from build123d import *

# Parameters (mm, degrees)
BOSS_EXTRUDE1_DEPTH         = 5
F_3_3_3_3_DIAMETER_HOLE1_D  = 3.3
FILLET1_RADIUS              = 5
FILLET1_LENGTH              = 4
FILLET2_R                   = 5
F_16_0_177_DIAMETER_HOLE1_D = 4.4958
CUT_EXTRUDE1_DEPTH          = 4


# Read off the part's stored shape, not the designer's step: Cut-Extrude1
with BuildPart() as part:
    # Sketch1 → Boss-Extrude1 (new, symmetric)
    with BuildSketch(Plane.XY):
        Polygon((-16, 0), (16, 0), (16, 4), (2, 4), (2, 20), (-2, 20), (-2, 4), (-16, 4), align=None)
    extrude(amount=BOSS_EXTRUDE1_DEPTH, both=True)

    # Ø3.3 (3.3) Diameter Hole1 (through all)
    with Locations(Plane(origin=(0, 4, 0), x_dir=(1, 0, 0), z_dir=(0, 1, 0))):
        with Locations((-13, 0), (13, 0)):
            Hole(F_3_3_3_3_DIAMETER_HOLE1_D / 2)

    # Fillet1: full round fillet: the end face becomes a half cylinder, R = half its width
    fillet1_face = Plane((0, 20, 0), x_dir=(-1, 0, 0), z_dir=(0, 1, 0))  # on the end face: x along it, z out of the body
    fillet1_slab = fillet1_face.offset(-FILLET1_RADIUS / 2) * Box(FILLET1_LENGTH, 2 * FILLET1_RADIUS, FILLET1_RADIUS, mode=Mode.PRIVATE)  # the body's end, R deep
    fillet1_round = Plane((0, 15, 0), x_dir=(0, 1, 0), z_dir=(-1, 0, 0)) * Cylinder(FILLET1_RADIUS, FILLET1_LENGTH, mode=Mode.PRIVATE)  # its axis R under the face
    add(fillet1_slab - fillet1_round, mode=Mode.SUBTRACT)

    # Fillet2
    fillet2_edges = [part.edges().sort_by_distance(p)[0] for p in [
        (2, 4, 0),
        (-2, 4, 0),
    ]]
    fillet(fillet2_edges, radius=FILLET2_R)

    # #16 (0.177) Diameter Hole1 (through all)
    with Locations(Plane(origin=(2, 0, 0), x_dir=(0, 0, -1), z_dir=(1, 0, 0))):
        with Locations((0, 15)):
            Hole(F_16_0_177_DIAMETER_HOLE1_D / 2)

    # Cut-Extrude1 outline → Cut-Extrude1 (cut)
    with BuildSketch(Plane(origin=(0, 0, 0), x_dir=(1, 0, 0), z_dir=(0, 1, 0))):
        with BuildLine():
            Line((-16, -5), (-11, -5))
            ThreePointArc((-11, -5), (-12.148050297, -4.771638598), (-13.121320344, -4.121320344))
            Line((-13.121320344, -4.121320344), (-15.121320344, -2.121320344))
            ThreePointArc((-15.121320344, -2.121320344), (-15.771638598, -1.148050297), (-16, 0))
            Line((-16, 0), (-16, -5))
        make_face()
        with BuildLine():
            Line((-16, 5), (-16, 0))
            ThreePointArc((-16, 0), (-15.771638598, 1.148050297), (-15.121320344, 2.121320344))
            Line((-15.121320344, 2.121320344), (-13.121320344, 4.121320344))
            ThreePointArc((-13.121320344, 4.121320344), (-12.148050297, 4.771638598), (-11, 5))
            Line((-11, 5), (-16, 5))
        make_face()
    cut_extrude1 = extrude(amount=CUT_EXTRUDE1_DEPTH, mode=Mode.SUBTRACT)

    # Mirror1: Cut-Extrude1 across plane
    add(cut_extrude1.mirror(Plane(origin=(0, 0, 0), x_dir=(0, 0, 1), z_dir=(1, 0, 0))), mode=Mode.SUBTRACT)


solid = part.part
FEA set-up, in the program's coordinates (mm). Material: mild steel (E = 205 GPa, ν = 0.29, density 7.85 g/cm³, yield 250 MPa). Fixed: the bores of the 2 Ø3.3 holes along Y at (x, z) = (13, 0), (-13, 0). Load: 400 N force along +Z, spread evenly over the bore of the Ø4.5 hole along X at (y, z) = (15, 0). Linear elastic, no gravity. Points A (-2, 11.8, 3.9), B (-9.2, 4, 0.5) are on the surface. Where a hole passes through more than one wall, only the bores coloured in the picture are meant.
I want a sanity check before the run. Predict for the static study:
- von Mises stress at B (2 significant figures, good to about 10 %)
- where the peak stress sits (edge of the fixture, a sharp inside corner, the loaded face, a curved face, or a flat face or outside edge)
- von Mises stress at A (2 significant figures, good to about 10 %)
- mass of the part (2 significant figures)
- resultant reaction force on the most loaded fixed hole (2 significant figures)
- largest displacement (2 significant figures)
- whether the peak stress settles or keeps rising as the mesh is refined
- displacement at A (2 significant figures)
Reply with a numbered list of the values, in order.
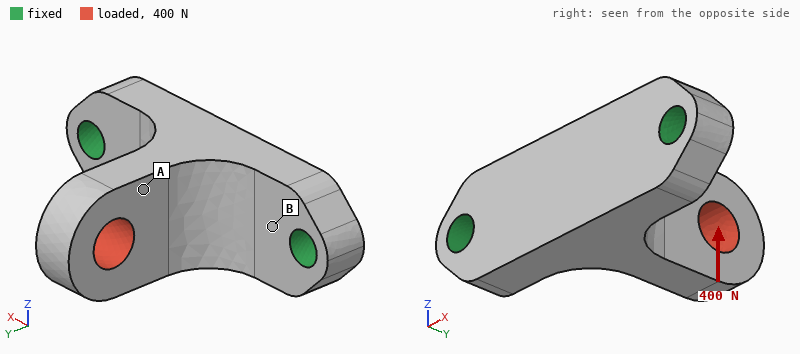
1. 99 MPa
2. edge of the fixture
3. 19 MPa
4. 14 g
5. 200 N
6. 37 µm
7. keeps rising
8. 21 µm
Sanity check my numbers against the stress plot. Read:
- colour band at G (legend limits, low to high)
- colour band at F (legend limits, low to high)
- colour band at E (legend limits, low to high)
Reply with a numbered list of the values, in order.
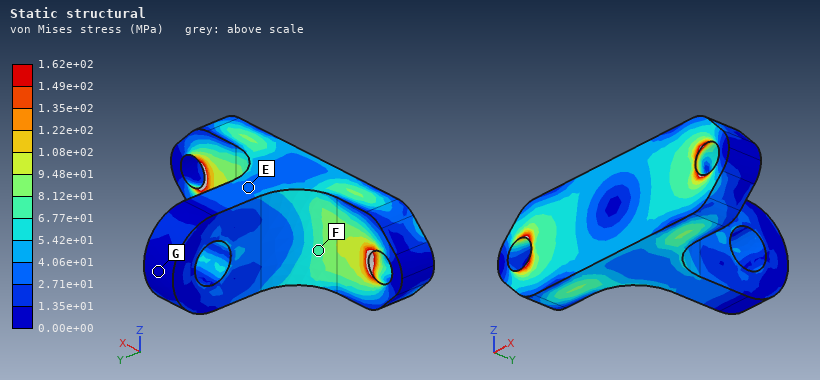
1. 0.00e+00 to 1.35e+01 MPa
2. 6.77e+01 to 8.12e+01 MPa
3. 2.71e+01 to 4.06e+01 MPa
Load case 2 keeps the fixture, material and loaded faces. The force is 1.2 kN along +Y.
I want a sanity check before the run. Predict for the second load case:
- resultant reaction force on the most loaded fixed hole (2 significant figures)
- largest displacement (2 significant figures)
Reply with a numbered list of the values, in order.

1. 650 N
2. 9.0 µm
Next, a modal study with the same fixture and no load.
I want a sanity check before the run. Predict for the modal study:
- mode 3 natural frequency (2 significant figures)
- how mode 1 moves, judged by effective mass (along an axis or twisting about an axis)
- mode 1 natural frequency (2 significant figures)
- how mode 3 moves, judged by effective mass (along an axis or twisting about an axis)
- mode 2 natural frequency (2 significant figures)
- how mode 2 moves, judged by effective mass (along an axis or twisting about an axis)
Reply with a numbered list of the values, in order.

1. 23 kHz
2. along Z
3. 11 kHz
4. along Y
5. 17 kHz
6. along X
